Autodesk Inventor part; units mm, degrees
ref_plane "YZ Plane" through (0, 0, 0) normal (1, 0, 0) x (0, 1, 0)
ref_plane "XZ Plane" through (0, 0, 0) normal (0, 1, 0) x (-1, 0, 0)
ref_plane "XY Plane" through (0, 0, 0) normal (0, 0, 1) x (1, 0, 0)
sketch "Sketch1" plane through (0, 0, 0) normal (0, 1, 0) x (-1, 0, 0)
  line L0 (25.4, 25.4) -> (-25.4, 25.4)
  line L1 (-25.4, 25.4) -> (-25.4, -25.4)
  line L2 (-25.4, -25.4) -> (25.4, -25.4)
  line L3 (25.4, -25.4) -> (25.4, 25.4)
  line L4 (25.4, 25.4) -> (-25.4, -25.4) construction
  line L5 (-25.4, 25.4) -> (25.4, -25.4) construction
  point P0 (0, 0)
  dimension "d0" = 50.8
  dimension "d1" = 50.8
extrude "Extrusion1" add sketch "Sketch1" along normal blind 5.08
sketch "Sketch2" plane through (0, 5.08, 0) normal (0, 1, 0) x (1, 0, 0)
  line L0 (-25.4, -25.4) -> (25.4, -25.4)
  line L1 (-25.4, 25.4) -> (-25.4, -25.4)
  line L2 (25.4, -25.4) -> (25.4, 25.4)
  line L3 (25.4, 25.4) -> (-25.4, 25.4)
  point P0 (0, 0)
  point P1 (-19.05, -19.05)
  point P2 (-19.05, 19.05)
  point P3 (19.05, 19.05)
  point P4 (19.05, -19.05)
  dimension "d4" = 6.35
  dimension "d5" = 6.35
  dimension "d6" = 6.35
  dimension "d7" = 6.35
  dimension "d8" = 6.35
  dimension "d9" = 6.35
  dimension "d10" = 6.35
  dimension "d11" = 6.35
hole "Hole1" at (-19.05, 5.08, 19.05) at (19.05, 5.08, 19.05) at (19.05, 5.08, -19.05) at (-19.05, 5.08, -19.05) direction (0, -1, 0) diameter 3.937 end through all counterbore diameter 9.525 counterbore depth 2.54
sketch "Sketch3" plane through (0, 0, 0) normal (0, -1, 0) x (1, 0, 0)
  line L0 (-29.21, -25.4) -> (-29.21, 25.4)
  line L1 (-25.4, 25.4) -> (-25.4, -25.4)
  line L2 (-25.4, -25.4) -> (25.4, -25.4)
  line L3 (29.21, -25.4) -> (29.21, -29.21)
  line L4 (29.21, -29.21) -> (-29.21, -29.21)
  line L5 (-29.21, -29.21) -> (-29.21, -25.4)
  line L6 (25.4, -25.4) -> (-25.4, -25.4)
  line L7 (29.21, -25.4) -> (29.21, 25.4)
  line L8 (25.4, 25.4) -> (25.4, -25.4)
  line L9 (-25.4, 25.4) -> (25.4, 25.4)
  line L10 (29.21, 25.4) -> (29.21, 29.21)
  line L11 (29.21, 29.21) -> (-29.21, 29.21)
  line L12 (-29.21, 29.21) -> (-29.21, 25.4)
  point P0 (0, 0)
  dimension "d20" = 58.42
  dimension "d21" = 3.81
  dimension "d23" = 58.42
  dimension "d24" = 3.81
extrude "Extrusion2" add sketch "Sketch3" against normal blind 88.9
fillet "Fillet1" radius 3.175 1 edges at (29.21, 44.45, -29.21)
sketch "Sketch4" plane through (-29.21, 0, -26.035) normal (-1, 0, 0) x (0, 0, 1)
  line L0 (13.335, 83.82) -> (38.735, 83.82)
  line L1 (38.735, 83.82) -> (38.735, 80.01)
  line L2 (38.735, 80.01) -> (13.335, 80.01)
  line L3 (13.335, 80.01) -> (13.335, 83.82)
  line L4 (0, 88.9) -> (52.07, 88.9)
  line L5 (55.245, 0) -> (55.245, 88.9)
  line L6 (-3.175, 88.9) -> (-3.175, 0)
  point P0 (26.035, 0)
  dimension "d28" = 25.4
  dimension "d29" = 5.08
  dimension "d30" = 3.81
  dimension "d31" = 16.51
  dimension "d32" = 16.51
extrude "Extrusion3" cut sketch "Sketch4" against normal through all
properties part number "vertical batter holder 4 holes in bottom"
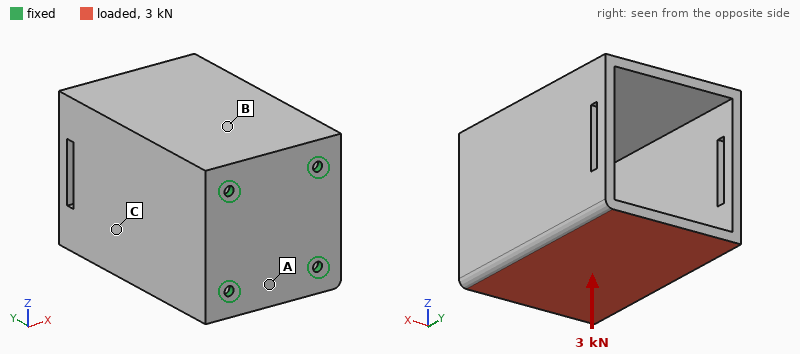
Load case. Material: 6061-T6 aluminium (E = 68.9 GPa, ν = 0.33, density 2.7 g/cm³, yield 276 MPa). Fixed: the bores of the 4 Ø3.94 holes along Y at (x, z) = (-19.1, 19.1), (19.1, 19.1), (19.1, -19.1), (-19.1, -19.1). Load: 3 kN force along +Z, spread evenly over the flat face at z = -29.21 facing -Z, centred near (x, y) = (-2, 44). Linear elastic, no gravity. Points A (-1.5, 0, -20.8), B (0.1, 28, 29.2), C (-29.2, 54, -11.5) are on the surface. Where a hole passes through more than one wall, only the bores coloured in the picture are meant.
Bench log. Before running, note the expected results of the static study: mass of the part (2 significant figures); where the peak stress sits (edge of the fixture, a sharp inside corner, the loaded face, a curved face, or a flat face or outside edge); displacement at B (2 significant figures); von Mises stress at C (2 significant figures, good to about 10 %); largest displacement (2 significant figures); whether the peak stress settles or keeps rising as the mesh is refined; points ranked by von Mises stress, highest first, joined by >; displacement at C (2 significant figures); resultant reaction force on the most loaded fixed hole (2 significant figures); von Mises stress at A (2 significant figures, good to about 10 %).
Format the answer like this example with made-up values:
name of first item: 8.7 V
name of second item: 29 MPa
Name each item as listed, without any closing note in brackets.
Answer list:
mass of the part: 230 g
where the peak stress sits: edge of the fixture
displacement at B: 0.038 mm
von Mises stress at C: 16 MPa
largest displacement: 0.22 mm
whether the peak stress settles or keeps rising as the mesh is refined: keeps rising
points ranked by von Mises stress, highest first, joined by >: A > C > B
displacement at C: 0.072 mm
resultant reaction force on the most loaded fixed hole: 1.9 kN
von Mises stress at A: 22 MPa
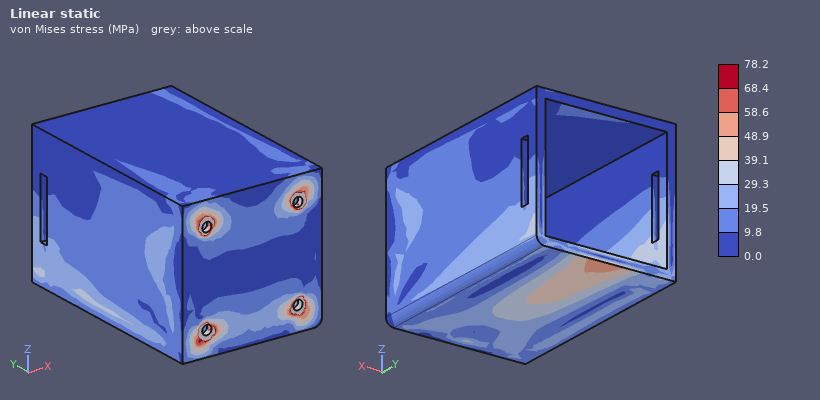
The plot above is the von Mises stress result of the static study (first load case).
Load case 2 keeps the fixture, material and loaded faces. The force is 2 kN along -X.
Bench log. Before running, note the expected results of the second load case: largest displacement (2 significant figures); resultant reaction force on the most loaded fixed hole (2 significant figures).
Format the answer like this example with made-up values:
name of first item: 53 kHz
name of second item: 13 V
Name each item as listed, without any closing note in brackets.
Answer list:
largest displacement: 0.11 mm
resultant reaction force on the most loaded fixed hole: 1.9 kN
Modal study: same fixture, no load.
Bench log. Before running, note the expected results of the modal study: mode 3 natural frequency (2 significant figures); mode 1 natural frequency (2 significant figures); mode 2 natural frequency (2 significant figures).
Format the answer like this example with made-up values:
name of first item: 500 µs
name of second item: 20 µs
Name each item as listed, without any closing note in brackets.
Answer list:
mode 3 natural frequency: 2500 Hz
mode 1 natural frequency: 2200 Hz
mode 2 natural frequency: 2200 Hz
